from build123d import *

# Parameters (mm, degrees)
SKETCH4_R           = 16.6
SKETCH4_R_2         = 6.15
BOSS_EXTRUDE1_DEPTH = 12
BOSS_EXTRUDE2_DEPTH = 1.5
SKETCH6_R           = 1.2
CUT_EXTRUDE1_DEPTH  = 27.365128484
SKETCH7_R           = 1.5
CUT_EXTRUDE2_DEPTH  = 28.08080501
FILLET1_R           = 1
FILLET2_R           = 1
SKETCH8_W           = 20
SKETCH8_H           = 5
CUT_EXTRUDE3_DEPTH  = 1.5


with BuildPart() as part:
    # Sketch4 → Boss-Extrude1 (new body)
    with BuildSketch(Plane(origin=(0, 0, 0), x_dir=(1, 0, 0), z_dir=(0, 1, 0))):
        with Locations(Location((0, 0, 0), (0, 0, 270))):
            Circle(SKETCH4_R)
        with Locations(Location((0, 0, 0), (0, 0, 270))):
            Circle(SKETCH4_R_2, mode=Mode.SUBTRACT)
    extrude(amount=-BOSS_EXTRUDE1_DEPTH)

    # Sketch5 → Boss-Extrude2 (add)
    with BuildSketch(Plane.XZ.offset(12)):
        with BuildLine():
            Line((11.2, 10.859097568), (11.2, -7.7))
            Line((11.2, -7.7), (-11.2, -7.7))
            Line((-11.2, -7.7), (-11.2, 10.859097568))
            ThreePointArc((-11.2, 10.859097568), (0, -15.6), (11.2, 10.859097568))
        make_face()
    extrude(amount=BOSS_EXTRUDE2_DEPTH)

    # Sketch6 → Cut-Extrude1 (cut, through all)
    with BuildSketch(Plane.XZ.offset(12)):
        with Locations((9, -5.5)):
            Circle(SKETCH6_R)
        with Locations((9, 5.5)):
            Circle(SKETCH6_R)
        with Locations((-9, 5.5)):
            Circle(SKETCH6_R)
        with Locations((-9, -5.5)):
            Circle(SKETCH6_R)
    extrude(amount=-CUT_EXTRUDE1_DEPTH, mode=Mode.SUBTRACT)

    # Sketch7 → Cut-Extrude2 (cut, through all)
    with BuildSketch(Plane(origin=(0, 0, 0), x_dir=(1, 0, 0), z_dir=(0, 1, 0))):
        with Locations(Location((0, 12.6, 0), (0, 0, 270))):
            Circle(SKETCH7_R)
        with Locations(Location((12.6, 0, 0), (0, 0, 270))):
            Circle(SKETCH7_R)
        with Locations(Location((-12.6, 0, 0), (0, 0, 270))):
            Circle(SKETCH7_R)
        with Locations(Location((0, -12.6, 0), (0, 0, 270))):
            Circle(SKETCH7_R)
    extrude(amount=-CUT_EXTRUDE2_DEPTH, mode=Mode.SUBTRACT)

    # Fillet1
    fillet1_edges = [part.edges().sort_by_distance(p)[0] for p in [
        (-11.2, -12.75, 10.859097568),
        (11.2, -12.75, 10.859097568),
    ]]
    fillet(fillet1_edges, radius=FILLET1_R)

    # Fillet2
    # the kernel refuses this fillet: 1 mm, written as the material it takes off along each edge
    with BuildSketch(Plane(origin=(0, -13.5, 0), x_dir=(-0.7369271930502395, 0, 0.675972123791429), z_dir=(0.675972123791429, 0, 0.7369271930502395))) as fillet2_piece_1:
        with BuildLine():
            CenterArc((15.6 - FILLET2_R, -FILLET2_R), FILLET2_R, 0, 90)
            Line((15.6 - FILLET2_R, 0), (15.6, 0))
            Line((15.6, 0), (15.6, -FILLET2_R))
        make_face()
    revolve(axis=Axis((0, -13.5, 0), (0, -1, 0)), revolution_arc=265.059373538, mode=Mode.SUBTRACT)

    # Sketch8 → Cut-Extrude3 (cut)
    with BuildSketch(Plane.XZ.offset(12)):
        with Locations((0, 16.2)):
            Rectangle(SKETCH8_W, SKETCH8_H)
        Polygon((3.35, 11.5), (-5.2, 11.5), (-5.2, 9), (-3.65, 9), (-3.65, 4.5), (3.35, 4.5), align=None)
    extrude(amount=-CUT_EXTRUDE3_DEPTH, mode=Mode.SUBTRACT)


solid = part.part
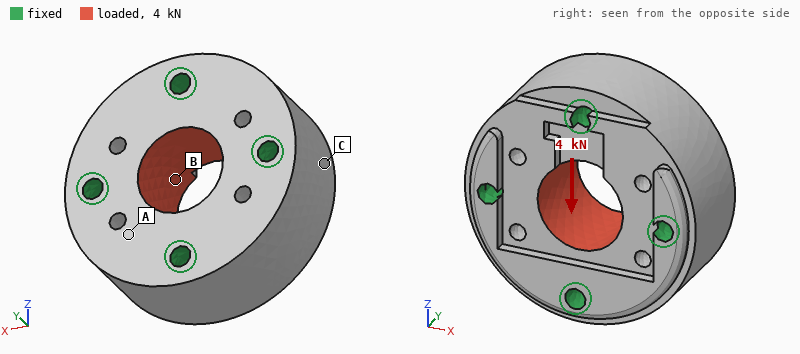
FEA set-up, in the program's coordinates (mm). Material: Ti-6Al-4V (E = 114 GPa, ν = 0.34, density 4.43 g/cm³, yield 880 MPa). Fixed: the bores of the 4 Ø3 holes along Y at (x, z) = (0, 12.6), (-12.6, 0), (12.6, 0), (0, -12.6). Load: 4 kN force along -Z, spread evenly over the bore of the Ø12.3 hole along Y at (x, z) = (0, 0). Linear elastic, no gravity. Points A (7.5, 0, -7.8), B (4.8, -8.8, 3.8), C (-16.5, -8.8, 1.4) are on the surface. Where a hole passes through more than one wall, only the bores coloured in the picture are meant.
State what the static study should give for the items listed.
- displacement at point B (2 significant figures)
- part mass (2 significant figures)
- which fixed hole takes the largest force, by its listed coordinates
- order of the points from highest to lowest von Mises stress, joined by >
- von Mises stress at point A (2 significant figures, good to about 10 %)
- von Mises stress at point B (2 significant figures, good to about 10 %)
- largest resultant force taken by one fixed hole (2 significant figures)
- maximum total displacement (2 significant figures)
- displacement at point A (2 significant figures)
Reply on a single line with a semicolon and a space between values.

1.0 µm; 38 g; (0, -12.6); B > A > C; 4.4 MPa; 13 MPa; 1.2 kN; 1.1 µm; 0.73 µm
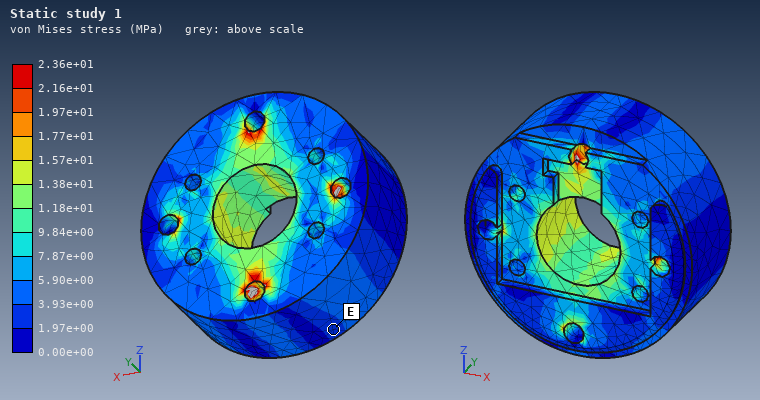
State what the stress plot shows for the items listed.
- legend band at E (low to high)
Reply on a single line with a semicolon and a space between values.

1.97e+00 to 3.93e+00 MPa
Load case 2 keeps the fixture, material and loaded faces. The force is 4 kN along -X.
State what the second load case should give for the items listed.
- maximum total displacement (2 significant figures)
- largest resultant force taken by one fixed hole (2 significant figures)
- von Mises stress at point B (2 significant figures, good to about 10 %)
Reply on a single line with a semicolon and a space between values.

1.1 µm; 1.1 kN; 12 MPa
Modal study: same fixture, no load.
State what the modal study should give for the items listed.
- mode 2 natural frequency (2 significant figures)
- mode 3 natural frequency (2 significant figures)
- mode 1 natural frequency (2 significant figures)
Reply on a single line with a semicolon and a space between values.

66 kHz; 66 kHz; 63 kHz
